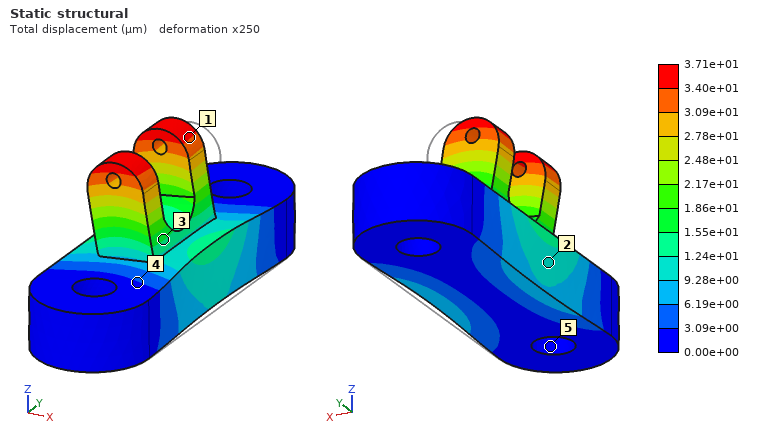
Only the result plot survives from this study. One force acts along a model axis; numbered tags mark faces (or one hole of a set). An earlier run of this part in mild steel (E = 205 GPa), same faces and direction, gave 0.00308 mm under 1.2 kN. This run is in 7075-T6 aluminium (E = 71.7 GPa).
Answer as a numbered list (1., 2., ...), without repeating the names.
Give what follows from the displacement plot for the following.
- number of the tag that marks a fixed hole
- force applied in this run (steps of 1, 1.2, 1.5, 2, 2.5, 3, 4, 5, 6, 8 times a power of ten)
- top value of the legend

1. 5
2. 5 kN
3. 3.71e+01 µm
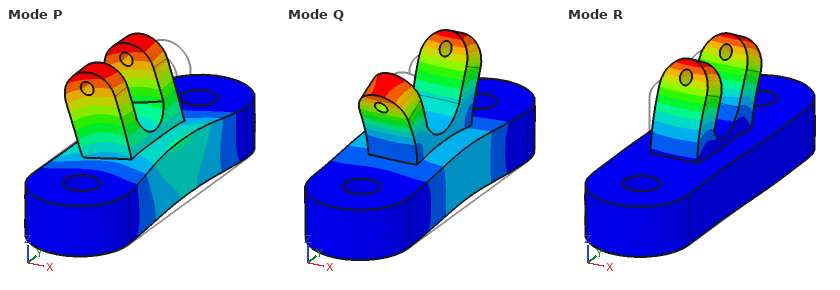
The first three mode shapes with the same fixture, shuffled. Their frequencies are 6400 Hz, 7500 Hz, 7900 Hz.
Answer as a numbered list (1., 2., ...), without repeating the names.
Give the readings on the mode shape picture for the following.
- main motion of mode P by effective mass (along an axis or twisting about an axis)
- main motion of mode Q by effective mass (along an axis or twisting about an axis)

1. along X
2. along Z
